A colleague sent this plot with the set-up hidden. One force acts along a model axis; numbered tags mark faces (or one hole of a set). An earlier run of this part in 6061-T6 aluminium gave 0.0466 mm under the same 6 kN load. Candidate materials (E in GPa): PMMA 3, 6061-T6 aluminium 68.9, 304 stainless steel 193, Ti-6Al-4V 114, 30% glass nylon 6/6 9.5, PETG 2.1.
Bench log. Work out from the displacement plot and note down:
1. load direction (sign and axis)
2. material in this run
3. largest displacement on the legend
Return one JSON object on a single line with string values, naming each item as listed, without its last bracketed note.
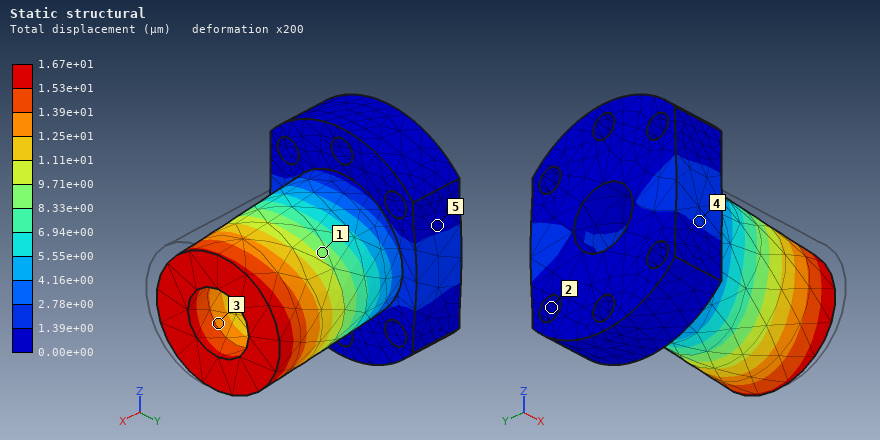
{"load direction": "+Y", "material in this run": "304 stainless steel", "largest displacement on the legend": "1.67e+01 µm"}
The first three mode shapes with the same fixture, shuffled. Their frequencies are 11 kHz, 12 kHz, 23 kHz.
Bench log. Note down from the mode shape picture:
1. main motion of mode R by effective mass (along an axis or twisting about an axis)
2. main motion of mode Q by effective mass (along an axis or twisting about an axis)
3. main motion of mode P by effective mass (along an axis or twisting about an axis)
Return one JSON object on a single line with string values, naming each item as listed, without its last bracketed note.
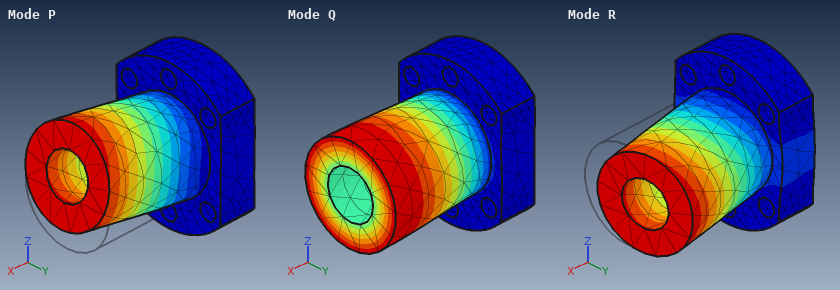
{"main motion of mode R by effective mass": "along Y", "main motion of mode Q by effective mass": "twisting about X", "main motion of mode P by effective mass": "along Z"}
